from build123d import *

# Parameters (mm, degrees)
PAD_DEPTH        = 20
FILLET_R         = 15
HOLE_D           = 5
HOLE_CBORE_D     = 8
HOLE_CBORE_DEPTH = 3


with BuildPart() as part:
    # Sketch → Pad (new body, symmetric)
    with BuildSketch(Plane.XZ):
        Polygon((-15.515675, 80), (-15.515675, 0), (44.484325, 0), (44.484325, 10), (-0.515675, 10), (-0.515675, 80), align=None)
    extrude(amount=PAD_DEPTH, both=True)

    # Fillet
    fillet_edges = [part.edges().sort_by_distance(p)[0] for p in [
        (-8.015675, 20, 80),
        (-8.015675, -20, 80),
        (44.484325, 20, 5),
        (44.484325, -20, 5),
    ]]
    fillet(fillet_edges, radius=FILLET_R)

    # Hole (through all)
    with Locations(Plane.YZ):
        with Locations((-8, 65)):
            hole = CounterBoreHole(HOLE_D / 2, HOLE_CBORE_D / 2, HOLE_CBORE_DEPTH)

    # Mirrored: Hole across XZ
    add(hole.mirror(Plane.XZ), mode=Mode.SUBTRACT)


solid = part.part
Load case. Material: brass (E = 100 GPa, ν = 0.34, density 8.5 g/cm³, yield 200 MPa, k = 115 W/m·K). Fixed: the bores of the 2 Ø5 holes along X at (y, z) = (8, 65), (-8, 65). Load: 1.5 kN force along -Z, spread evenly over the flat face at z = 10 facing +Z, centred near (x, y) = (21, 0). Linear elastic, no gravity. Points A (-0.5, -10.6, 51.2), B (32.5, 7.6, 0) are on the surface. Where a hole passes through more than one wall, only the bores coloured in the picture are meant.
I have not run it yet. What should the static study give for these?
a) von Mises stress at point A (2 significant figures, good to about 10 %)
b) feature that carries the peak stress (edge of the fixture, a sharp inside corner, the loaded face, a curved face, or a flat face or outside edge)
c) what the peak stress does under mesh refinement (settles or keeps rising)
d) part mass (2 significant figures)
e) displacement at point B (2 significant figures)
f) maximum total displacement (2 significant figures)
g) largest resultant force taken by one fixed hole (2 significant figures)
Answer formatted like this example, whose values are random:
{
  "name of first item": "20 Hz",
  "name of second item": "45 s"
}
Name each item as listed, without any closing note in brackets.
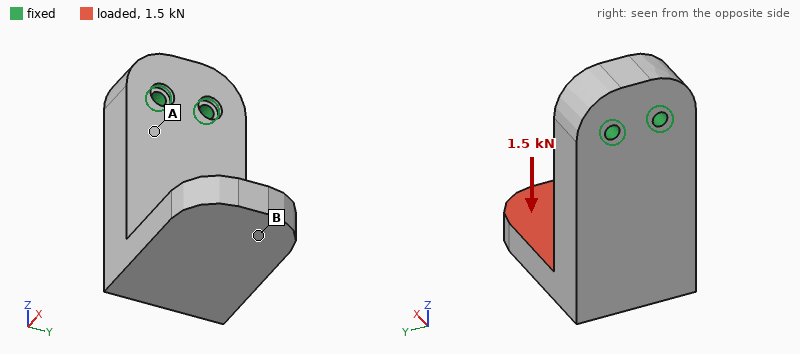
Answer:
{
  "von Mises stress at point A": "31 MPa",
  "feature that carries the peak stress": "edge of the fixture",
  "what the peak stress does under mesh refinement": "keeps rising",
  "part mass": "530 g",
  "displacement at point B": "0.17 mm",
  "maximum total displacement": "0.22 mm",
  "largest resultant force taken by one fixed hole": "750 N"
}
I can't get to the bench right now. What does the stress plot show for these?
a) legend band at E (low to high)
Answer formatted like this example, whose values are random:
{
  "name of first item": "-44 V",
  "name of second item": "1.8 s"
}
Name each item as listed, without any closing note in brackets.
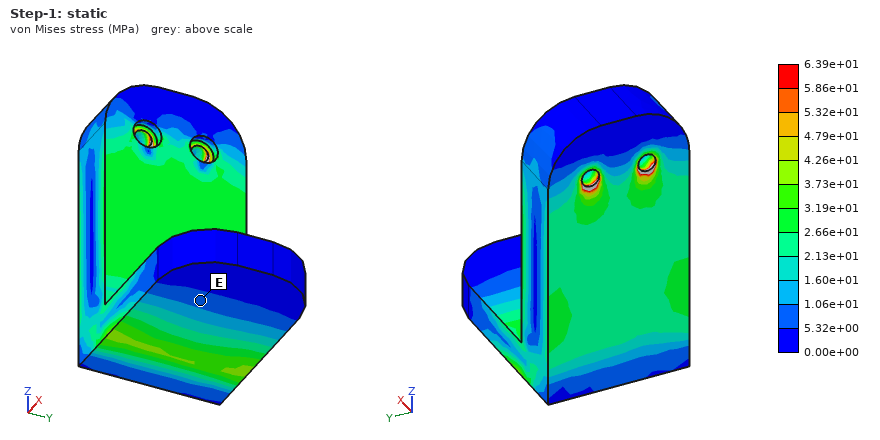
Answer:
{
  "legend band at E": "5.32e+00 to 1.06e+01 MPa"
}
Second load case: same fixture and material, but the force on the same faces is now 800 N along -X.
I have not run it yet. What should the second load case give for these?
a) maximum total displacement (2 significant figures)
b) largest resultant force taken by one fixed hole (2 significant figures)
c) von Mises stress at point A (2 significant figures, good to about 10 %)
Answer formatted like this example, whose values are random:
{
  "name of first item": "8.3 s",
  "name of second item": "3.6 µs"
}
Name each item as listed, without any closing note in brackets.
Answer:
{
  "maximum total displacement": "82 µm",
  "largest resultant force taken by one fixed hole": "400 N",
  "von Mises stress at point A": "21 MPa"
}
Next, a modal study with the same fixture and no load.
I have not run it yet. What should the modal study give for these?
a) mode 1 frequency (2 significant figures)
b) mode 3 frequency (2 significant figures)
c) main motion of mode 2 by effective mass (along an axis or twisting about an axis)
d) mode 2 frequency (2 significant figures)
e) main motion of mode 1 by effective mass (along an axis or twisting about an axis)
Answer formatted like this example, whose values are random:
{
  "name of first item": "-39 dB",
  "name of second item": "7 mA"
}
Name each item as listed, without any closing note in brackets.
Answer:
{
  "mode 1 frequency": "960 Hz",
  "mode 3 frequency": "2300 Hz",
  "main motion of mode 2 by effective mass": "along Y",
  "mode 2 frequency": "1600 Hz",
  "main motion of mode 1 by effective mass": "along X"
}
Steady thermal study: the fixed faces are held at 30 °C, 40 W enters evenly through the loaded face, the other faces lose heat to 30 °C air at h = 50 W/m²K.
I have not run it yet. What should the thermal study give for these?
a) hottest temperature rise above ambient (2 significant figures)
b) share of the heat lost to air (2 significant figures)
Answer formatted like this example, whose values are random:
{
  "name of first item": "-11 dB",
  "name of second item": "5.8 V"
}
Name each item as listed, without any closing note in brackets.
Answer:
{
  "hottest temperature rise above ambient": "45 K",
  "share of the heat lost to air": "28 %"
}
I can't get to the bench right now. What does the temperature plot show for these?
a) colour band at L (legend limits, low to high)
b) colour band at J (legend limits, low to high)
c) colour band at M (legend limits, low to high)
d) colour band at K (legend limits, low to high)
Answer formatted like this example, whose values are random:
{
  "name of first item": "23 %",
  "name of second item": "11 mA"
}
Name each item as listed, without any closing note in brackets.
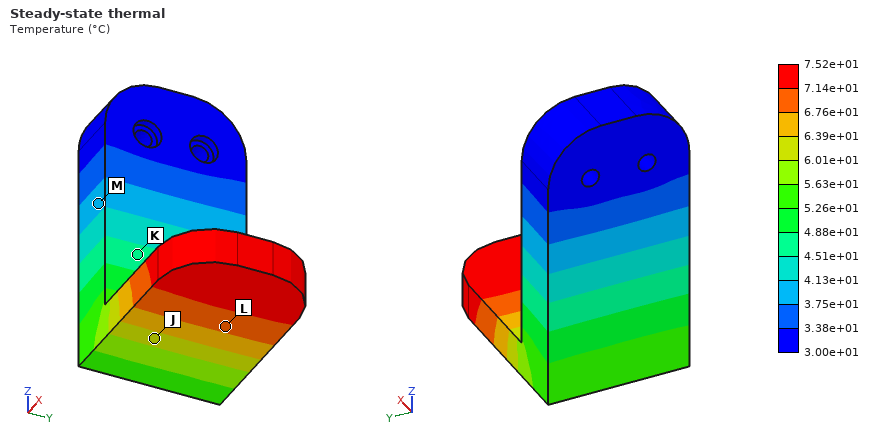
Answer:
{
  "colour band at L": "6.76e+01 to 7.14e+01 °C",
  "colour band at J": "6.01e+01 to 6.39e+01 °C",
  "colour band at M": "3.75e+01 to 4.13e+01 °C",
  "colour band at K": "4.51e+01 to 4.88e+01 °C"
}
